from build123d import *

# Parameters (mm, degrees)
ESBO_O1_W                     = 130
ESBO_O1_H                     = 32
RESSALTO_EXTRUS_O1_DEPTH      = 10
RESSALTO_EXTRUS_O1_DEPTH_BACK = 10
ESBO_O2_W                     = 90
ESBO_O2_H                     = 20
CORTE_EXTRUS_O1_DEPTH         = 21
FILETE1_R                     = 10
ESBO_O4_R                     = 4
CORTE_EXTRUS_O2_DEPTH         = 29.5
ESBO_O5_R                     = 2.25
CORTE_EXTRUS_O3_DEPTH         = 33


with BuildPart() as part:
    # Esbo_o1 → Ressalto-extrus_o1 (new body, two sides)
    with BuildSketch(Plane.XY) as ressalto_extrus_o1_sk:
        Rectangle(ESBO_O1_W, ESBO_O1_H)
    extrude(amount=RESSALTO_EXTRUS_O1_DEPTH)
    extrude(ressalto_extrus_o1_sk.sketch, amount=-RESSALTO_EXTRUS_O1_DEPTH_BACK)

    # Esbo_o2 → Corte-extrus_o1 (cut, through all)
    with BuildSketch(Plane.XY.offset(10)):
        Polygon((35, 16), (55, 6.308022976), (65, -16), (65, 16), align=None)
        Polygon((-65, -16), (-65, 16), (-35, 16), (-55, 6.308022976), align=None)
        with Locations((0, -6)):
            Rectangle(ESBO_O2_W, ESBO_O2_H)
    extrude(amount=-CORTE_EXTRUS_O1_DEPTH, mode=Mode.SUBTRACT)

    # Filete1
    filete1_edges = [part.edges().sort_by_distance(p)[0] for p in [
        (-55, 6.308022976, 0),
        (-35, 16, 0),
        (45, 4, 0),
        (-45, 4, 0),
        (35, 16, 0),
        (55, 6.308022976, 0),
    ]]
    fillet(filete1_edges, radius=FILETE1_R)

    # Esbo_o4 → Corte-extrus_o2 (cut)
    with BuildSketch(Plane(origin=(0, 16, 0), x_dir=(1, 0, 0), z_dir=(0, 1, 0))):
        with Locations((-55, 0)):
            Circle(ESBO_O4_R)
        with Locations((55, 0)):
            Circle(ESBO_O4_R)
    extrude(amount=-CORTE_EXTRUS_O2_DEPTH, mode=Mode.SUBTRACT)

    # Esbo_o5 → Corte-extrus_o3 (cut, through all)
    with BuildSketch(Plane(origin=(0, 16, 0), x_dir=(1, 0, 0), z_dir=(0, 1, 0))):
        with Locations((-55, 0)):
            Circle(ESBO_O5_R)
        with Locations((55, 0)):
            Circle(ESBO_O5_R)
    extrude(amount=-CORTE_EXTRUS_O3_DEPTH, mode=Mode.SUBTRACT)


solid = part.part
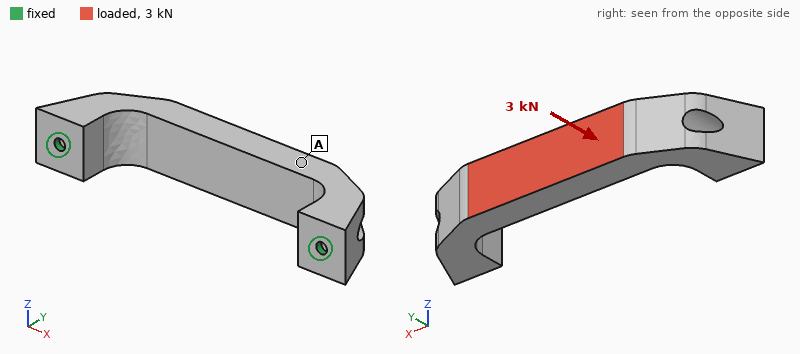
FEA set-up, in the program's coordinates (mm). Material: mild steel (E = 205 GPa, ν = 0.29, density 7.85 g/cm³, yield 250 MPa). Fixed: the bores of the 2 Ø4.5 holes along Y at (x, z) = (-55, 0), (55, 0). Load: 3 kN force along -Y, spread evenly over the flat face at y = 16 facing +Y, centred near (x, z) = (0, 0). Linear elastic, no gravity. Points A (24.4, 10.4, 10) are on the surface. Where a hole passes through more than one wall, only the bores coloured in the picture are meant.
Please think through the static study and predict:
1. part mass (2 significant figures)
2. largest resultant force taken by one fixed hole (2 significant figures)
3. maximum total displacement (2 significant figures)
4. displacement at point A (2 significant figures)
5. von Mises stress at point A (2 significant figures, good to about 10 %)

270 g
2.1 kN
27 µm
17 µm
17 MPa
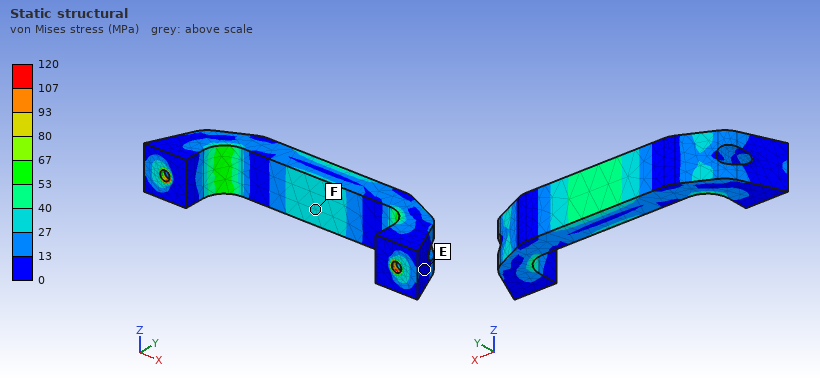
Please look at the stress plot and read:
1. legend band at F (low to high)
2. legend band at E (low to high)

27 to 40 MPa
0 to 13 MPa
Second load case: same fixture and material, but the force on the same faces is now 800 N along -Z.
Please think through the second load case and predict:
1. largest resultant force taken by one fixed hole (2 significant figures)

400 N
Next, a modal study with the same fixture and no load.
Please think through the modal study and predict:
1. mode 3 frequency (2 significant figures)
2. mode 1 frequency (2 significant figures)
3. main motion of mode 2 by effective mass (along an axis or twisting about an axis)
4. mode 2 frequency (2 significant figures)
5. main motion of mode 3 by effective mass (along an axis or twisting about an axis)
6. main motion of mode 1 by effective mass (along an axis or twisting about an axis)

4800 Hz
1500 Hz
along X
3800 Hz
twisting about Y
along Z
